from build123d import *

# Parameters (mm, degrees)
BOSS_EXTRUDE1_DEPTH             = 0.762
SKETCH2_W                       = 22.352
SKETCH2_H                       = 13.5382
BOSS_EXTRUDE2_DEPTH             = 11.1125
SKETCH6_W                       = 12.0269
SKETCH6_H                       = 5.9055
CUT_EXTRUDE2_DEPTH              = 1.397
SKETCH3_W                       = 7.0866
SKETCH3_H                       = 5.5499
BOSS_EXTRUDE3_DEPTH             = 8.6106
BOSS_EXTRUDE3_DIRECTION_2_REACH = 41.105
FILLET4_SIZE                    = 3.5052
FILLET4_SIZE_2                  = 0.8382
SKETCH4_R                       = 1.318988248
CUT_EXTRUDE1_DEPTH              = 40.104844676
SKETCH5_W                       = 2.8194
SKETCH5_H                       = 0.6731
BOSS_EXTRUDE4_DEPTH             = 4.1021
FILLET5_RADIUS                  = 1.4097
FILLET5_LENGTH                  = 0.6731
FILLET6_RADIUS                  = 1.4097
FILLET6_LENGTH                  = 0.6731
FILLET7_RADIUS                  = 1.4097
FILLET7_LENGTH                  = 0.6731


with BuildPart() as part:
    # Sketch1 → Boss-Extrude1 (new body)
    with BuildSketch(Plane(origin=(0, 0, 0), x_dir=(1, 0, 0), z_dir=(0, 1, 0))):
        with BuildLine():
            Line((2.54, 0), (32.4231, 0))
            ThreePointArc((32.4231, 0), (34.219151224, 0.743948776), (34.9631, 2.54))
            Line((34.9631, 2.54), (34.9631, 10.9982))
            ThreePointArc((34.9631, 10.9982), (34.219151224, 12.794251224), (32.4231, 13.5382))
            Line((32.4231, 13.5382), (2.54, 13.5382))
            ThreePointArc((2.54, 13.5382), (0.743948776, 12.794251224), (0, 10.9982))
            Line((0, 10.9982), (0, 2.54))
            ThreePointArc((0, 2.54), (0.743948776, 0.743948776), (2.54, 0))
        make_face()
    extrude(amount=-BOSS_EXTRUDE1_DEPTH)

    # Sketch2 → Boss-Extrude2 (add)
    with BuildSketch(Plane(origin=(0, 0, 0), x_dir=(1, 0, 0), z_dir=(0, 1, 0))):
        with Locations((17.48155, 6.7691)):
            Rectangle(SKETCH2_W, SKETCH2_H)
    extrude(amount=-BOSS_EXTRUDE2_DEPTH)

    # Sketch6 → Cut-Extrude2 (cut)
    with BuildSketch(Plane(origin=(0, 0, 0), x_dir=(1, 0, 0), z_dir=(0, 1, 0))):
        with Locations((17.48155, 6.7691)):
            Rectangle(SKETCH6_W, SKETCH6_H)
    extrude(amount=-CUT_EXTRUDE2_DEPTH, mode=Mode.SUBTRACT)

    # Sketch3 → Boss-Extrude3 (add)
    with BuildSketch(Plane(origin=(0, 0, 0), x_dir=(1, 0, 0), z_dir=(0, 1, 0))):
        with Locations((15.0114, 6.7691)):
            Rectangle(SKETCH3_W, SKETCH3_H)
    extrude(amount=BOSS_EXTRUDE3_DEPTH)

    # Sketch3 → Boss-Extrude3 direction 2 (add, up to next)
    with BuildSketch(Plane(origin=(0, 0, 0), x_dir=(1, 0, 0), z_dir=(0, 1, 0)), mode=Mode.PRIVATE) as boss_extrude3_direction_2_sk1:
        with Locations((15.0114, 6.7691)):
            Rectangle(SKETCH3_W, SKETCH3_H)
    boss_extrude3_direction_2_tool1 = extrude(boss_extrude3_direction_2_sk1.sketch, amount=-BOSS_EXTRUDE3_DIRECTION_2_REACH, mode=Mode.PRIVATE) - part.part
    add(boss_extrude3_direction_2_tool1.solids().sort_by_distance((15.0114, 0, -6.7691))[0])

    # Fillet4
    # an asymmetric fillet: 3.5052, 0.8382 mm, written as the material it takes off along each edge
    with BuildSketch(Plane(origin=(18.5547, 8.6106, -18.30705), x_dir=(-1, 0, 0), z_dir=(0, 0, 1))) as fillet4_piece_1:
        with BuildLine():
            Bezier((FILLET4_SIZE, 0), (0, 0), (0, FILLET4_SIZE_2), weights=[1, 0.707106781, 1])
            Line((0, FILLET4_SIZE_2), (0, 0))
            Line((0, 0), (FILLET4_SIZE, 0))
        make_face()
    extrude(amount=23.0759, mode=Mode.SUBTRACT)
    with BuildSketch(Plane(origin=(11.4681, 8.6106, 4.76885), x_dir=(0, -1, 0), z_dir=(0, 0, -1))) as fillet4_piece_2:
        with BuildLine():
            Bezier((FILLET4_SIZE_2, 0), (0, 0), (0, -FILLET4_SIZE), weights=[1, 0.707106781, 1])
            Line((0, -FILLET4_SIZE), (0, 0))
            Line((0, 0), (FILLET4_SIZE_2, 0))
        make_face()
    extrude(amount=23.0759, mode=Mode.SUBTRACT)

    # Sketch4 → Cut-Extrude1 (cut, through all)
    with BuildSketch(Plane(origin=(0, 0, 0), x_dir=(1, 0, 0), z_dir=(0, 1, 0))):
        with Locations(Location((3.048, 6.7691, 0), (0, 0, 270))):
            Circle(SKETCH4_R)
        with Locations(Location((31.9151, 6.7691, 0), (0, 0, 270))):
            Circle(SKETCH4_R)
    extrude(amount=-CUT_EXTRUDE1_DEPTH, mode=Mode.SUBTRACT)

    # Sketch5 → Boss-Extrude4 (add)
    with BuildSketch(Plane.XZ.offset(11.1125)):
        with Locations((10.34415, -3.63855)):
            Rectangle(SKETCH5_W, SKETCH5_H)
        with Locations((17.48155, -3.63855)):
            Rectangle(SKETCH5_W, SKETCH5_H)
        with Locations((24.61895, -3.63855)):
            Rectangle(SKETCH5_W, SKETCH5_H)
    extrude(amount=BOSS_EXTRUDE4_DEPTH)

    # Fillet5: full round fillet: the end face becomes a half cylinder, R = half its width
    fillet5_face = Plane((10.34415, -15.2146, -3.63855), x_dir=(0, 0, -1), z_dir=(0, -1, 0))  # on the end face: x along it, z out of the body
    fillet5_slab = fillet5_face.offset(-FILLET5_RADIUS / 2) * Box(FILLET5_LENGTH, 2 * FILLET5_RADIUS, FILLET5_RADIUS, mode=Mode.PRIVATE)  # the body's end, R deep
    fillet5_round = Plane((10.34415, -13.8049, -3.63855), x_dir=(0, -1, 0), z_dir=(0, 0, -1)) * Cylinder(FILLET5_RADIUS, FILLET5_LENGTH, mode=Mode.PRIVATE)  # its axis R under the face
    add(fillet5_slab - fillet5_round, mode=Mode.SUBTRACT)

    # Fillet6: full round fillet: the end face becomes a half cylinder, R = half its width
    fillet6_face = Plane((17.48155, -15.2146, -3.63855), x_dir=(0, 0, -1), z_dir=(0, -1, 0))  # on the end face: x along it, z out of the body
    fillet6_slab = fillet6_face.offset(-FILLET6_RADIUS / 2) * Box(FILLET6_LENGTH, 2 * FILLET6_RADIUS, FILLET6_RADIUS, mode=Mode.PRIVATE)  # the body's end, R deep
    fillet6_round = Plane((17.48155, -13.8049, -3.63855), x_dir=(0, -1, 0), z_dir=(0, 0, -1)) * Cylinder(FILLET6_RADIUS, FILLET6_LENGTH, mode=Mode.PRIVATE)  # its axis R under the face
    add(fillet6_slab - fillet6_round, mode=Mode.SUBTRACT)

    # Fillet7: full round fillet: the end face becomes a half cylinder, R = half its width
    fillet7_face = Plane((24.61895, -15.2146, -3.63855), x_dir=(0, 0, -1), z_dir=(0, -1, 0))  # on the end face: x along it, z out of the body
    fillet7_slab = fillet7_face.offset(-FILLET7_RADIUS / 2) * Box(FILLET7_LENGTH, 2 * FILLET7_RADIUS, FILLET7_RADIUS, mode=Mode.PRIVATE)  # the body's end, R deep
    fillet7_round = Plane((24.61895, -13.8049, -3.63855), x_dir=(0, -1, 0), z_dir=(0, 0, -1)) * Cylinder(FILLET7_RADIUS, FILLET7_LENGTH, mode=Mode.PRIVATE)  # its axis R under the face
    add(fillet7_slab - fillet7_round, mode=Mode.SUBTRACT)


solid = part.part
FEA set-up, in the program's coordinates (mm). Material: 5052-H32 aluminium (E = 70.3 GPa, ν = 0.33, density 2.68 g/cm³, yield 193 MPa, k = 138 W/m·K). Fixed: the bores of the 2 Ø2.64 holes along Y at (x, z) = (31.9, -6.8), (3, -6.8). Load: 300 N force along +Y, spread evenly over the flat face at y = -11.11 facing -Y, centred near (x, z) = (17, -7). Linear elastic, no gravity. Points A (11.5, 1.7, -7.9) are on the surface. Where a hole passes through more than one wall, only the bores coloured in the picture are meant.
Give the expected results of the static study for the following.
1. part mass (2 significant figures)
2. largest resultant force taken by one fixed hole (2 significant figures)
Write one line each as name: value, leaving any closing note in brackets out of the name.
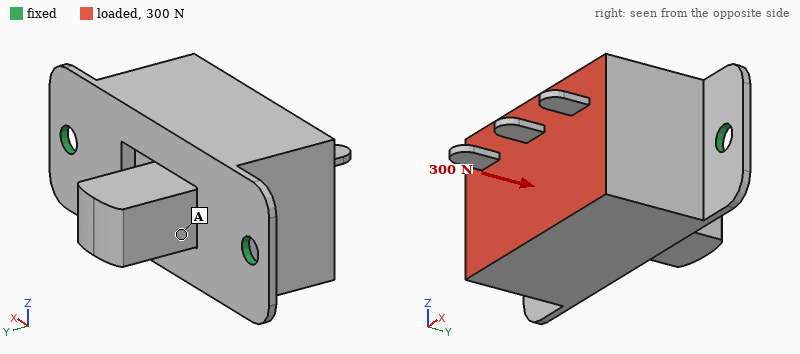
part mass: 10 g
largest resultant force taken by one fixed hole: 170 N
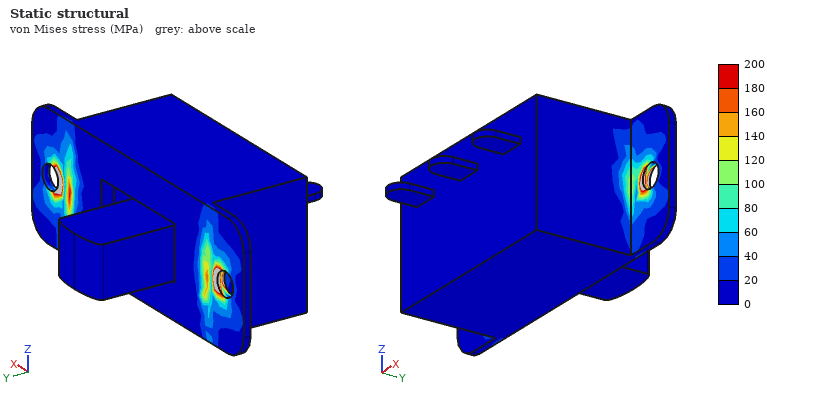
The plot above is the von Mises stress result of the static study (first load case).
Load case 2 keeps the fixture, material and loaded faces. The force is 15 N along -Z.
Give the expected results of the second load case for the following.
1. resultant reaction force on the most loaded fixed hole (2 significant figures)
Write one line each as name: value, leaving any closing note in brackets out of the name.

resultant reaction force on the most loaded fixed hole: 7.5 N
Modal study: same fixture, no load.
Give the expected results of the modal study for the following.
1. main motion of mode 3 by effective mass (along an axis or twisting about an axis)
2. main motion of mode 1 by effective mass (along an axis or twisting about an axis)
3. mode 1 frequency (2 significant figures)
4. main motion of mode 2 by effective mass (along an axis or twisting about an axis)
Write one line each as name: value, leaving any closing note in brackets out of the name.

main motion of mode 3 by effective mass: along X
main motion of mode 1 by effective mass: along Z
mode 1 frequency: 1800 Hz
main motion of mode 2 by effective mass: along Y
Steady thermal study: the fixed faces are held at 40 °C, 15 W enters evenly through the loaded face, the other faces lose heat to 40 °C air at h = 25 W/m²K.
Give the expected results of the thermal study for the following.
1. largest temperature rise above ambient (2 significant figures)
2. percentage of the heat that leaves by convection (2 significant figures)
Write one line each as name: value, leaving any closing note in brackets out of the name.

largest temperature rise above ambient: 30 K
percentage of the heat that leaves by convection: 7.1 %
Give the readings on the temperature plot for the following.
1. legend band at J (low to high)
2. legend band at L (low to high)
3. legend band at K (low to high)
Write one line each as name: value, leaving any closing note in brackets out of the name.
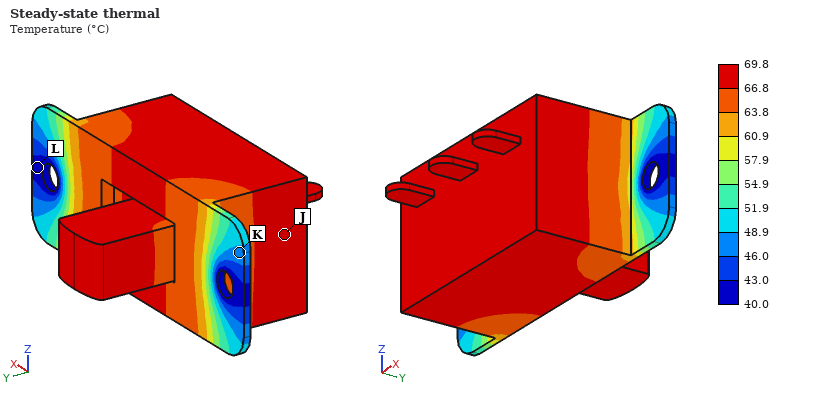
legend band at J: 66.8 to 69.8 °C
legend band at L: 40.0 to 43.0 °C
legend band at K: 46.0 to 48.9 °C
